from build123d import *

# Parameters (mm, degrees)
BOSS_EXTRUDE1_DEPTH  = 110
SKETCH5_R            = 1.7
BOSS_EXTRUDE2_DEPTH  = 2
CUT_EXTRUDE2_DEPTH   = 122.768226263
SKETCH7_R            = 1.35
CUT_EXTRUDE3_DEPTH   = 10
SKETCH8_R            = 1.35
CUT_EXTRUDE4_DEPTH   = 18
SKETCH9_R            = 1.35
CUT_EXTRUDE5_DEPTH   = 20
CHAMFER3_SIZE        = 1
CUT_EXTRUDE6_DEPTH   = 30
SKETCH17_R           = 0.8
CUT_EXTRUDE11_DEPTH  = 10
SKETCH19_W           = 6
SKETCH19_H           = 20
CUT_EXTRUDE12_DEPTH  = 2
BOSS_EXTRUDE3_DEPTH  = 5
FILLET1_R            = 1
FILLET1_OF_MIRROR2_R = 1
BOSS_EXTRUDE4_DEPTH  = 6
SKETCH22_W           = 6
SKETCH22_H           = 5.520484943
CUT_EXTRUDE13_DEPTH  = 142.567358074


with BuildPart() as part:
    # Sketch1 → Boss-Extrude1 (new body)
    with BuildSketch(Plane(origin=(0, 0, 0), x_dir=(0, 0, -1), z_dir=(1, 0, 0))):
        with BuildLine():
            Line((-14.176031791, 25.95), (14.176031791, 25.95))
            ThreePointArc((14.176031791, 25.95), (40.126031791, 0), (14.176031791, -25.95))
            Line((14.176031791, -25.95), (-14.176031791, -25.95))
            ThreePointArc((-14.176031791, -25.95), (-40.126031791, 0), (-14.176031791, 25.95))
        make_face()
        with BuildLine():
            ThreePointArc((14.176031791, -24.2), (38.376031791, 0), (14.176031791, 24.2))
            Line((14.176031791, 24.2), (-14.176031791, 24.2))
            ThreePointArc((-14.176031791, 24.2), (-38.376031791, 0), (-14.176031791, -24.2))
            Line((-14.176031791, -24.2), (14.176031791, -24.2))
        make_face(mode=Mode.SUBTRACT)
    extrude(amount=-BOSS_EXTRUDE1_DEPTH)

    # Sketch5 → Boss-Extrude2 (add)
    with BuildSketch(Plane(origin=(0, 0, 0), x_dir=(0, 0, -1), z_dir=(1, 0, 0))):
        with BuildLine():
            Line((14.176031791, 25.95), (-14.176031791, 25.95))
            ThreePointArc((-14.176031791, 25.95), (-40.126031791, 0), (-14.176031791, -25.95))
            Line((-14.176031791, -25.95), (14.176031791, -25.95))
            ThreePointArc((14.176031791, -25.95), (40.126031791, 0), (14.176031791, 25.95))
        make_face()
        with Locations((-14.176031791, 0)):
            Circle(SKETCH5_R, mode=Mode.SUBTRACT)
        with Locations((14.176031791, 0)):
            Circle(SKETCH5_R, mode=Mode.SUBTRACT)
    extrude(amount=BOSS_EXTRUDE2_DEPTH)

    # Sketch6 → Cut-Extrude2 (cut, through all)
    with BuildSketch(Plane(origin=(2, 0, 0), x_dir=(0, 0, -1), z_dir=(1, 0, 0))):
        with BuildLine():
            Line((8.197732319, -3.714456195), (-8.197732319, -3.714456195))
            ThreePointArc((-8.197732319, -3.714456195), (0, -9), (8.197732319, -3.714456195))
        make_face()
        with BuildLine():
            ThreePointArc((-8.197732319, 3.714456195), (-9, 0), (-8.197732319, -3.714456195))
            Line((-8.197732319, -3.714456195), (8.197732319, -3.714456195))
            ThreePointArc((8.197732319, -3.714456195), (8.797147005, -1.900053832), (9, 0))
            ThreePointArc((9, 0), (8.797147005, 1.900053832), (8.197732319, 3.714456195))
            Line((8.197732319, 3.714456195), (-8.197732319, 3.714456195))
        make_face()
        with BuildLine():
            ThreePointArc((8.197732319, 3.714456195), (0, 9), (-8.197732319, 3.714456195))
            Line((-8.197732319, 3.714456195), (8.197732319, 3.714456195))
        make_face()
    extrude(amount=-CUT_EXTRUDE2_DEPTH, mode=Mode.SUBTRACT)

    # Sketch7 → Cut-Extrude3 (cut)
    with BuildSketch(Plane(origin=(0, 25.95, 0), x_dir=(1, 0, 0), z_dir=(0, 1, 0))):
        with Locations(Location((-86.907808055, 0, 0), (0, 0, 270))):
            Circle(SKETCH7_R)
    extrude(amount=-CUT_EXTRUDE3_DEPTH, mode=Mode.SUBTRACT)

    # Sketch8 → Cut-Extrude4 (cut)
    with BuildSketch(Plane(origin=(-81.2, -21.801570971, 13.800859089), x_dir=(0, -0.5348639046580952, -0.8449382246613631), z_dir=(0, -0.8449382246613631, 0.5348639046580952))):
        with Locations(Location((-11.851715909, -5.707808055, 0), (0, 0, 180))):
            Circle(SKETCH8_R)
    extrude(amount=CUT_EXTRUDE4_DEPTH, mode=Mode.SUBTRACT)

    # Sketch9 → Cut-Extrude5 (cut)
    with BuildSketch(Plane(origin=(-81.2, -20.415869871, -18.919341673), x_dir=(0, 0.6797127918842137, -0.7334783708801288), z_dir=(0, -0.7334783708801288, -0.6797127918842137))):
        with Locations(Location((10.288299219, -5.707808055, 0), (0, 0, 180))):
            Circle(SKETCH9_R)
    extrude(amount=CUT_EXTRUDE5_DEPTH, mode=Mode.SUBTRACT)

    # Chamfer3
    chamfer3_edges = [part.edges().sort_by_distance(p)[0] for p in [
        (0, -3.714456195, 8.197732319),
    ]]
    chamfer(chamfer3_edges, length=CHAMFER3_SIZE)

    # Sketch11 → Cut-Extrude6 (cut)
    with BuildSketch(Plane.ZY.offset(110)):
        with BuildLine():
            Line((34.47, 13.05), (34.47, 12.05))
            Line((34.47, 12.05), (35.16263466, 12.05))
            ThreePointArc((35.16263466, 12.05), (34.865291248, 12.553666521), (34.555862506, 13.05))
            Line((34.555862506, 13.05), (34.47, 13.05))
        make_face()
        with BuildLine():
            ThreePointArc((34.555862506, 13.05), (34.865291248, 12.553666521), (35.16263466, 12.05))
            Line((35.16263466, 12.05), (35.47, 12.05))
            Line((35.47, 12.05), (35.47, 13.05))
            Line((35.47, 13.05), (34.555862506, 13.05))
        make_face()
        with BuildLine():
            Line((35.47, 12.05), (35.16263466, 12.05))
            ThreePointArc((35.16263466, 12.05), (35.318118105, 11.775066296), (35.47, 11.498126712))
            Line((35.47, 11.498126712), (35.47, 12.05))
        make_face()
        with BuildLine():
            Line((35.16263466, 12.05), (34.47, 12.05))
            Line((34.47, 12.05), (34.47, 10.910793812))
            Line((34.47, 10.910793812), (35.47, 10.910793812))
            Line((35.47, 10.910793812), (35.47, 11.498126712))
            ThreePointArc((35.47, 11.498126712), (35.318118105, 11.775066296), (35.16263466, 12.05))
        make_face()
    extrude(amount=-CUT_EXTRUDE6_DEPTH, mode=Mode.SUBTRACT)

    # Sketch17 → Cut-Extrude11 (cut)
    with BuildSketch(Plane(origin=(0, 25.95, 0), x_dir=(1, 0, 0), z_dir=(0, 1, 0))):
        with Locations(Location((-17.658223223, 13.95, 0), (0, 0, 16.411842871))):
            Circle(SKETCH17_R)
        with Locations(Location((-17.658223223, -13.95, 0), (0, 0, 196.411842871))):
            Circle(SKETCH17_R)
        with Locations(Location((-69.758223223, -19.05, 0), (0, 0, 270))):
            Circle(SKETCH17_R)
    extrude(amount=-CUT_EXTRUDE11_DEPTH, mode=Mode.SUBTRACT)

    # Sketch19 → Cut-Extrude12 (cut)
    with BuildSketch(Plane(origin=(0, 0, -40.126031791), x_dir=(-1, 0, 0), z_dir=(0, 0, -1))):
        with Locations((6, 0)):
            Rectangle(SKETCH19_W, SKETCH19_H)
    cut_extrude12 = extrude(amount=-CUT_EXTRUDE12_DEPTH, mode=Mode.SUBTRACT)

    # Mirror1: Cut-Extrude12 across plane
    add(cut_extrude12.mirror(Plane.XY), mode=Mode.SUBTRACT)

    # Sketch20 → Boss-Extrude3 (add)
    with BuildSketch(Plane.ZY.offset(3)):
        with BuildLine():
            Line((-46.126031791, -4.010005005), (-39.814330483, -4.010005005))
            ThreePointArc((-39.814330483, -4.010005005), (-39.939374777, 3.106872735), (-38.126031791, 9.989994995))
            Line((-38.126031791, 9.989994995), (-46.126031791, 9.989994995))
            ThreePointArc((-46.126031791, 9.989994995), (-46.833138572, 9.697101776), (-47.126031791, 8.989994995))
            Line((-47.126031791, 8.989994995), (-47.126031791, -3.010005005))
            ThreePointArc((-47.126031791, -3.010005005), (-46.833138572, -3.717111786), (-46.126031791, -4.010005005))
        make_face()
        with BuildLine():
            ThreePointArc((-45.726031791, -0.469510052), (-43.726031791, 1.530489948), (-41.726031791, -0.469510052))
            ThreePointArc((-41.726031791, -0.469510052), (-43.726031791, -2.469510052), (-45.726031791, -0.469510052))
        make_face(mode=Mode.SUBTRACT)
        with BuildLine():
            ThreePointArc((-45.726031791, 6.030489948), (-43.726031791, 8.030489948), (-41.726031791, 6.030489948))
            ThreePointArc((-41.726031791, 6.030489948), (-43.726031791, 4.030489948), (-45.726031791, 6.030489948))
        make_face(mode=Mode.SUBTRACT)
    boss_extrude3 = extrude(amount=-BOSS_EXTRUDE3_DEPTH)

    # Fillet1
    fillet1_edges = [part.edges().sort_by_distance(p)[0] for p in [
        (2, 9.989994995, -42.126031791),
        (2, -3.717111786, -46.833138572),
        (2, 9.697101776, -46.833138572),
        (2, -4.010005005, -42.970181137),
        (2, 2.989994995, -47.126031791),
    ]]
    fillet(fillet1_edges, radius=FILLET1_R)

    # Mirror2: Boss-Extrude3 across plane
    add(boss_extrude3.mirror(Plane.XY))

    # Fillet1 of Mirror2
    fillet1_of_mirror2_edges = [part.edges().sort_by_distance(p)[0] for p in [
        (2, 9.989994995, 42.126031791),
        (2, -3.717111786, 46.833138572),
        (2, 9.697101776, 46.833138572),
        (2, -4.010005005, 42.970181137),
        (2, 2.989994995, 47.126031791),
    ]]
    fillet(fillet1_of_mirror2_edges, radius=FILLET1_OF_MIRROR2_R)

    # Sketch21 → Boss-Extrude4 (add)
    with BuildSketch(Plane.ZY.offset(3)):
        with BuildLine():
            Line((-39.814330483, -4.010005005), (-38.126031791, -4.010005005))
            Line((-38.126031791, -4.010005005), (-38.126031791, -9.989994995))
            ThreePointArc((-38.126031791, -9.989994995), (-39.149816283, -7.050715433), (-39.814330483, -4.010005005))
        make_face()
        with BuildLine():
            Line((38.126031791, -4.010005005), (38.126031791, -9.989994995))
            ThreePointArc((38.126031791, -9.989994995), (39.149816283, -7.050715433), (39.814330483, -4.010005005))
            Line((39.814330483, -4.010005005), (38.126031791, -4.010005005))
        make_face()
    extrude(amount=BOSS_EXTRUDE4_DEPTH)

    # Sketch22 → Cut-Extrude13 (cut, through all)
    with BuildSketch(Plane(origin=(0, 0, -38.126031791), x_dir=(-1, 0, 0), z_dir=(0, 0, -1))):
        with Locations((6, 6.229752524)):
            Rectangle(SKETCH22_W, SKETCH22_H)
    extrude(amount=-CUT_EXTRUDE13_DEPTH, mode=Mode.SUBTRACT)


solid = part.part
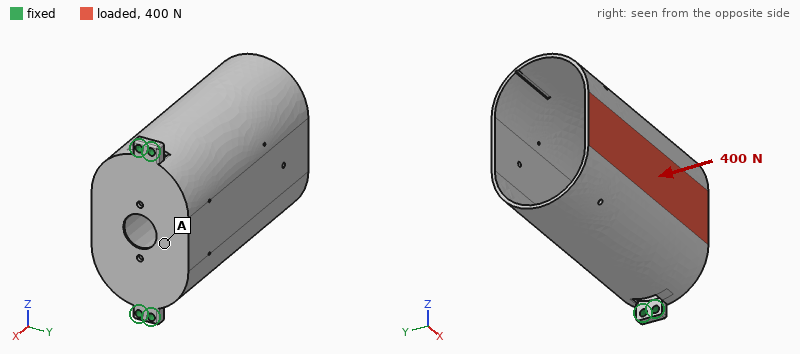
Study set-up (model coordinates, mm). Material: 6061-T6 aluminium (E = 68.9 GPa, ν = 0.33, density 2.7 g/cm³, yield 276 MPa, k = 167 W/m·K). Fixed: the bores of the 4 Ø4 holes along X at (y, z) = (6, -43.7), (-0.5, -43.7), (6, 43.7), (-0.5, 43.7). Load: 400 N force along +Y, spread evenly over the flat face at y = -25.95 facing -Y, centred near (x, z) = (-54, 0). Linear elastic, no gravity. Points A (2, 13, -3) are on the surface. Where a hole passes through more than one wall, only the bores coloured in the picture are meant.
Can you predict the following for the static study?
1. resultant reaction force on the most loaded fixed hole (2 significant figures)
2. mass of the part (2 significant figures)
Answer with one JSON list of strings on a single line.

["880 N", "130 g"]
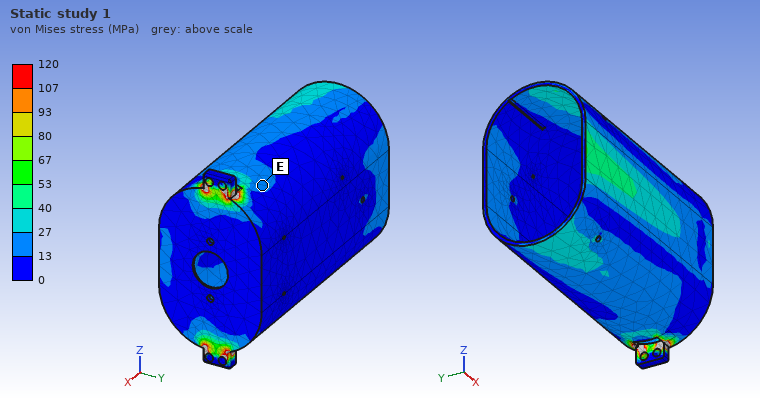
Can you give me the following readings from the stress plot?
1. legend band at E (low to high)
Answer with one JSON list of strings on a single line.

["13 to 27 MPa"]
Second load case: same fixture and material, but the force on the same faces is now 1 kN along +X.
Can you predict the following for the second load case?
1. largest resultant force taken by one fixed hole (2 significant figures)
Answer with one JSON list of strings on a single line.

["1.4 kN"]
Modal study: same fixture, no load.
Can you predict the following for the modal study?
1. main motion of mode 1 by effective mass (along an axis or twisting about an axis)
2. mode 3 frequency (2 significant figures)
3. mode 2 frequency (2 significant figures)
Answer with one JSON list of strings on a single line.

["along Y", "1100 Hz", "1000 Hz"]
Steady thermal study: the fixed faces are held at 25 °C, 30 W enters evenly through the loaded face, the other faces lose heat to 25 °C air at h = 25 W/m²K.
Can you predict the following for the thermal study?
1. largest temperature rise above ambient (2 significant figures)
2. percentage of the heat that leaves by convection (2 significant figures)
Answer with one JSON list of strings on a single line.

["31 K", "61 %"]
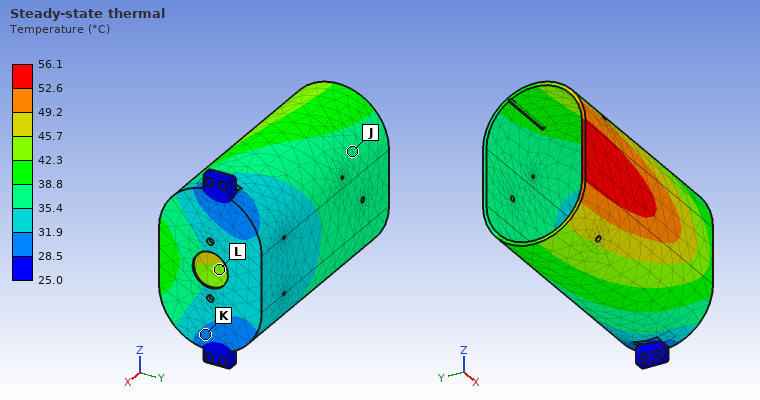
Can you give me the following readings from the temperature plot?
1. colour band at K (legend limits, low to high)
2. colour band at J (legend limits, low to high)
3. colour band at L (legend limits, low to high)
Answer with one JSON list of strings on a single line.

["28.5 to 31.9 °C", "35.4 to 38.8 °C", "42.3 to 45.7 °C"]
